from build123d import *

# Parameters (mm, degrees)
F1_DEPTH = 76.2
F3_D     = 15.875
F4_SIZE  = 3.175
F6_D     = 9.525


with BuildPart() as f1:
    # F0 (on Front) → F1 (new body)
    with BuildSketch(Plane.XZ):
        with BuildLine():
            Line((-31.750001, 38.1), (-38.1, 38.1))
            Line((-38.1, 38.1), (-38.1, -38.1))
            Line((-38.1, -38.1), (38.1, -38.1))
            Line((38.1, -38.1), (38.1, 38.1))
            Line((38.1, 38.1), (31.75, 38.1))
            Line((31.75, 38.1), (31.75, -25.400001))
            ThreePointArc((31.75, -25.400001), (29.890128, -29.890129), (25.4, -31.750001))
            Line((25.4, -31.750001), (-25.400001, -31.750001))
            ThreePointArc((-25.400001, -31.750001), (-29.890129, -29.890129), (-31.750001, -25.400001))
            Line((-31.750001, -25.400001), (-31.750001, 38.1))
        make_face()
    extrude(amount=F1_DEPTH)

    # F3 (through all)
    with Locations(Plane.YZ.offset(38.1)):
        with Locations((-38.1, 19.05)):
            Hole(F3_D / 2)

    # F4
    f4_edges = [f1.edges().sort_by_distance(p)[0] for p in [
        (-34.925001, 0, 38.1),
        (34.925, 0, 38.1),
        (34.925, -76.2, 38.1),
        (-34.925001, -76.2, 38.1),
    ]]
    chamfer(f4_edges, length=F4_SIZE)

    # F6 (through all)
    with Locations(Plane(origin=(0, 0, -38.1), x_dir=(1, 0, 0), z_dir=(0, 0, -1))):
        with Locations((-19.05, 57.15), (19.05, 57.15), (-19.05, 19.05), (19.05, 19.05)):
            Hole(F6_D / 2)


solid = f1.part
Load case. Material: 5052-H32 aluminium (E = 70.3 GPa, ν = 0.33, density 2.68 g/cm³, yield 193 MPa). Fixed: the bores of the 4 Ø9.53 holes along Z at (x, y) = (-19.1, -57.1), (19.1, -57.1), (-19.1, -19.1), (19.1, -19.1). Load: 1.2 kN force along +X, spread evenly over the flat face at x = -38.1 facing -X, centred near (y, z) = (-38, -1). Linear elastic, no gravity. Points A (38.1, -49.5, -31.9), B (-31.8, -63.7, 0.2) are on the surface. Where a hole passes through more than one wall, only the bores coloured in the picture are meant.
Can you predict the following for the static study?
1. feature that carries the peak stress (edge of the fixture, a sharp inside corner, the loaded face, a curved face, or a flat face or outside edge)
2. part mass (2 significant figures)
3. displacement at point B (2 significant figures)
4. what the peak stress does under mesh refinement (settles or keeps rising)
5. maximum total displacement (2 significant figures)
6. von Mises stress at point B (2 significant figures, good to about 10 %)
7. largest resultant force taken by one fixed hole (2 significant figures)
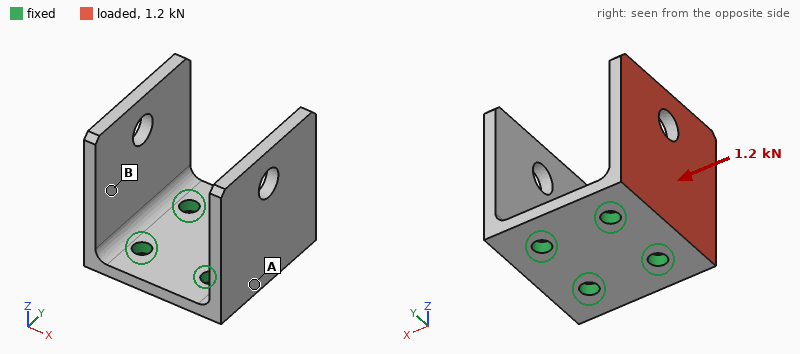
edge of the fixture
270 g
0.22 mm
keeps rising
0.61 mm
21 MPa
560 N
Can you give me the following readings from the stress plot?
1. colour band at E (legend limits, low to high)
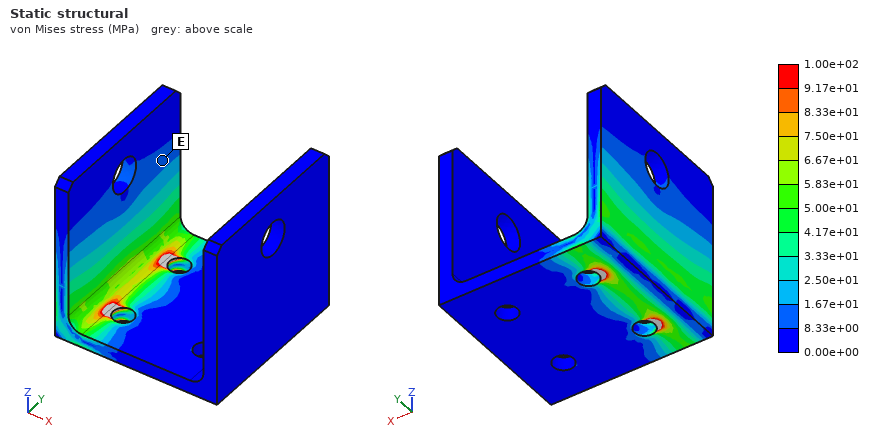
8.33e+00 to 1.67e+01 MPa
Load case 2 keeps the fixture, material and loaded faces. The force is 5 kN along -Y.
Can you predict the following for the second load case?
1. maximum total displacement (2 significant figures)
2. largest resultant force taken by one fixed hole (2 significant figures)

0.19 mm
4.9 kN
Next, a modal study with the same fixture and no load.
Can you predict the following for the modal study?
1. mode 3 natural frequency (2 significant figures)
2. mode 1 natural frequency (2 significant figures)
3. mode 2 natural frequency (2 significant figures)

2000 Hz
900 Hz
900 Hz
